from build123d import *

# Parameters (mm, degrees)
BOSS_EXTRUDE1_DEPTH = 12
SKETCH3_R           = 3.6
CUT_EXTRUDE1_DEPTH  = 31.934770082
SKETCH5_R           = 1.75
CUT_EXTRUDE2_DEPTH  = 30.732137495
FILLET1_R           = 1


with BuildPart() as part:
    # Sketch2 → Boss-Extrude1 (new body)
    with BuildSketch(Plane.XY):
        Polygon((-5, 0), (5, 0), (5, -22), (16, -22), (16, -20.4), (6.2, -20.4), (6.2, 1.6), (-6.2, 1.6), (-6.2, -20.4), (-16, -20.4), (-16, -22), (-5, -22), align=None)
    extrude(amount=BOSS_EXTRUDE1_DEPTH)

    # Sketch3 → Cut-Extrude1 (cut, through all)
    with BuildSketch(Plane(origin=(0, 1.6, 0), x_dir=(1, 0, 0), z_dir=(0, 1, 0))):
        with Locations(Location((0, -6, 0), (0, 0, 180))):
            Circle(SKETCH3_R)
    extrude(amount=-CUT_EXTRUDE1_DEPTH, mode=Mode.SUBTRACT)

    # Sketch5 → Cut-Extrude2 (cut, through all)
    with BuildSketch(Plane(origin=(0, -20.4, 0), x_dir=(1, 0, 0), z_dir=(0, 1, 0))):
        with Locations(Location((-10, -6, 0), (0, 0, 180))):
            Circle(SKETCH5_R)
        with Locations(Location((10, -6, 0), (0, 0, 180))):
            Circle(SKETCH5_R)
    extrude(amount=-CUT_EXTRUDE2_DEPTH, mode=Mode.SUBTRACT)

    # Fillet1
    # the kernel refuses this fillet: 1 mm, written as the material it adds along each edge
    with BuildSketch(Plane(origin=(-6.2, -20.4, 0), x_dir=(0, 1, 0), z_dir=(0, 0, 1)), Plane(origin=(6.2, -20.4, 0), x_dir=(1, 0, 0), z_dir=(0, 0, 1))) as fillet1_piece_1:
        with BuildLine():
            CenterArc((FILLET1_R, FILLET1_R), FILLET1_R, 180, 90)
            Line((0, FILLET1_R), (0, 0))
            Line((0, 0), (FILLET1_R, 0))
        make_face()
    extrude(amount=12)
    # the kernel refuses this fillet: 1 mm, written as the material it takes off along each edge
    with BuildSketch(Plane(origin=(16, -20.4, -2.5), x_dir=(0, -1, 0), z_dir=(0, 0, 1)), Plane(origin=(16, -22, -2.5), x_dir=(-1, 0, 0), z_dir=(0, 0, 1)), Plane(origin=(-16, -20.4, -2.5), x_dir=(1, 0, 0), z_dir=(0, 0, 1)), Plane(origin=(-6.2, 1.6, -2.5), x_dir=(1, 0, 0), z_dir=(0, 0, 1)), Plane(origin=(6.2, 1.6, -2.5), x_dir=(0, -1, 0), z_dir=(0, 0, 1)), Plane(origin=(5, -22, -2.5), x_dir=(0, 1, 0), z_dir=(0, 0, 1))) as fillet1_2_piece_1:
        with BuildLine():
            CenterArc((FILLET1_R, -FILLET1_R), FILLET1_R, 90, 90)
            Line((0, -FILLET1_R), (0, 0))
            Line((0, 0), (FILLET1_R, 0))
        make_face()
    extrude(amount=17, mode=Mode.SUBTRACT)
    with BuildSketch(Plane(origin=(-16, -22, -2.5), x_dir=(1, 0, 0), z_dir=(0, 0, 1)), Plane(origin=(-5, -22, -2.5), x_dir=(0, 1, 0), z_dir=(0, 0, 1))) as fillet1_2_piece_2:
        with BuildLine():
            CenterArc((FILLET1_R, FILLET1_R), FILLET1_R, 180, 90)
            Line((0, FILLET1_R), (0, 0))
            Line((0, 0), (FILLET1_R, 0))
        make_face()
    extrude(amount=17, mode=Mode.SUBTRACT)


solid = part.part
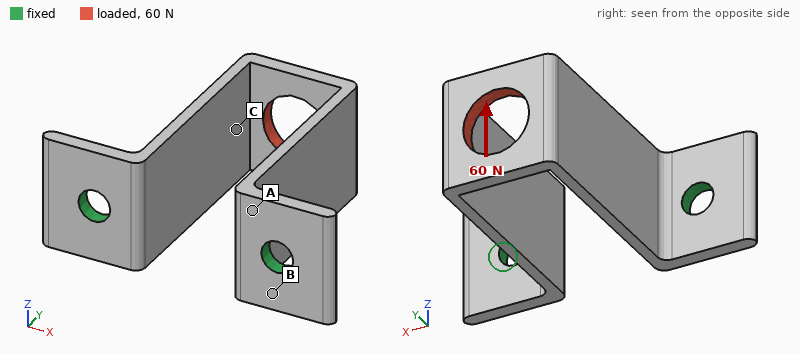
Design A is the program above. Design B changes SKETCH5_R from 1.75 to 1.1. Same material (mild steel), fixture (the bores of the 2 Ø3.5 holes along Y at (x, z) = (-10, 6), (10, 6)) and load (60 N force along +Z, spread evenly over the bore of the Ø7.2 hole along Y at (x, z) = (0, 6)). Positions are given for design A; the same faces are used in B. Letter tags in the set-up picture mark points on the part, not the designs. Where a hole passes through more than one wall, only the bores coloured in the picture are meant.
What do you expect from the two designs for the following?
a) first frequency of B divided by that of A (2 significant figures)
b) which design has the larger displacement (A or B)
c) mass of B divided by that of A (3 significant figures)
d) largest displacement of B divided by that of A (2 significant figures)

0.99
B
1.02
1.4
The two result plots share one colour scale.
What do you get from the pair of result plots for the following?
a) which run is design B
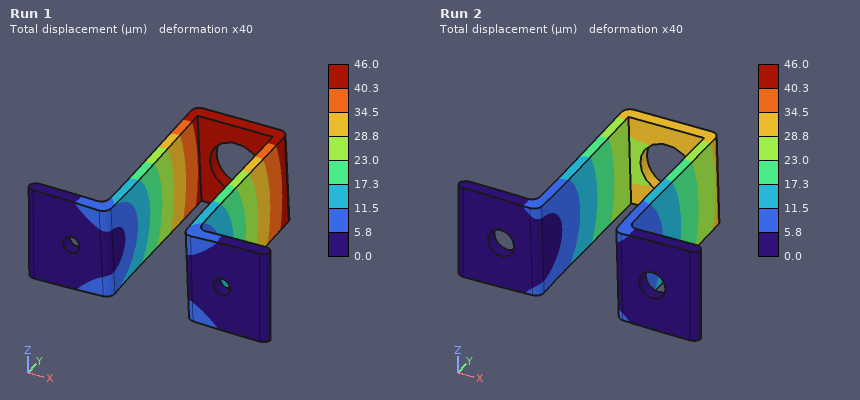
Run 1
